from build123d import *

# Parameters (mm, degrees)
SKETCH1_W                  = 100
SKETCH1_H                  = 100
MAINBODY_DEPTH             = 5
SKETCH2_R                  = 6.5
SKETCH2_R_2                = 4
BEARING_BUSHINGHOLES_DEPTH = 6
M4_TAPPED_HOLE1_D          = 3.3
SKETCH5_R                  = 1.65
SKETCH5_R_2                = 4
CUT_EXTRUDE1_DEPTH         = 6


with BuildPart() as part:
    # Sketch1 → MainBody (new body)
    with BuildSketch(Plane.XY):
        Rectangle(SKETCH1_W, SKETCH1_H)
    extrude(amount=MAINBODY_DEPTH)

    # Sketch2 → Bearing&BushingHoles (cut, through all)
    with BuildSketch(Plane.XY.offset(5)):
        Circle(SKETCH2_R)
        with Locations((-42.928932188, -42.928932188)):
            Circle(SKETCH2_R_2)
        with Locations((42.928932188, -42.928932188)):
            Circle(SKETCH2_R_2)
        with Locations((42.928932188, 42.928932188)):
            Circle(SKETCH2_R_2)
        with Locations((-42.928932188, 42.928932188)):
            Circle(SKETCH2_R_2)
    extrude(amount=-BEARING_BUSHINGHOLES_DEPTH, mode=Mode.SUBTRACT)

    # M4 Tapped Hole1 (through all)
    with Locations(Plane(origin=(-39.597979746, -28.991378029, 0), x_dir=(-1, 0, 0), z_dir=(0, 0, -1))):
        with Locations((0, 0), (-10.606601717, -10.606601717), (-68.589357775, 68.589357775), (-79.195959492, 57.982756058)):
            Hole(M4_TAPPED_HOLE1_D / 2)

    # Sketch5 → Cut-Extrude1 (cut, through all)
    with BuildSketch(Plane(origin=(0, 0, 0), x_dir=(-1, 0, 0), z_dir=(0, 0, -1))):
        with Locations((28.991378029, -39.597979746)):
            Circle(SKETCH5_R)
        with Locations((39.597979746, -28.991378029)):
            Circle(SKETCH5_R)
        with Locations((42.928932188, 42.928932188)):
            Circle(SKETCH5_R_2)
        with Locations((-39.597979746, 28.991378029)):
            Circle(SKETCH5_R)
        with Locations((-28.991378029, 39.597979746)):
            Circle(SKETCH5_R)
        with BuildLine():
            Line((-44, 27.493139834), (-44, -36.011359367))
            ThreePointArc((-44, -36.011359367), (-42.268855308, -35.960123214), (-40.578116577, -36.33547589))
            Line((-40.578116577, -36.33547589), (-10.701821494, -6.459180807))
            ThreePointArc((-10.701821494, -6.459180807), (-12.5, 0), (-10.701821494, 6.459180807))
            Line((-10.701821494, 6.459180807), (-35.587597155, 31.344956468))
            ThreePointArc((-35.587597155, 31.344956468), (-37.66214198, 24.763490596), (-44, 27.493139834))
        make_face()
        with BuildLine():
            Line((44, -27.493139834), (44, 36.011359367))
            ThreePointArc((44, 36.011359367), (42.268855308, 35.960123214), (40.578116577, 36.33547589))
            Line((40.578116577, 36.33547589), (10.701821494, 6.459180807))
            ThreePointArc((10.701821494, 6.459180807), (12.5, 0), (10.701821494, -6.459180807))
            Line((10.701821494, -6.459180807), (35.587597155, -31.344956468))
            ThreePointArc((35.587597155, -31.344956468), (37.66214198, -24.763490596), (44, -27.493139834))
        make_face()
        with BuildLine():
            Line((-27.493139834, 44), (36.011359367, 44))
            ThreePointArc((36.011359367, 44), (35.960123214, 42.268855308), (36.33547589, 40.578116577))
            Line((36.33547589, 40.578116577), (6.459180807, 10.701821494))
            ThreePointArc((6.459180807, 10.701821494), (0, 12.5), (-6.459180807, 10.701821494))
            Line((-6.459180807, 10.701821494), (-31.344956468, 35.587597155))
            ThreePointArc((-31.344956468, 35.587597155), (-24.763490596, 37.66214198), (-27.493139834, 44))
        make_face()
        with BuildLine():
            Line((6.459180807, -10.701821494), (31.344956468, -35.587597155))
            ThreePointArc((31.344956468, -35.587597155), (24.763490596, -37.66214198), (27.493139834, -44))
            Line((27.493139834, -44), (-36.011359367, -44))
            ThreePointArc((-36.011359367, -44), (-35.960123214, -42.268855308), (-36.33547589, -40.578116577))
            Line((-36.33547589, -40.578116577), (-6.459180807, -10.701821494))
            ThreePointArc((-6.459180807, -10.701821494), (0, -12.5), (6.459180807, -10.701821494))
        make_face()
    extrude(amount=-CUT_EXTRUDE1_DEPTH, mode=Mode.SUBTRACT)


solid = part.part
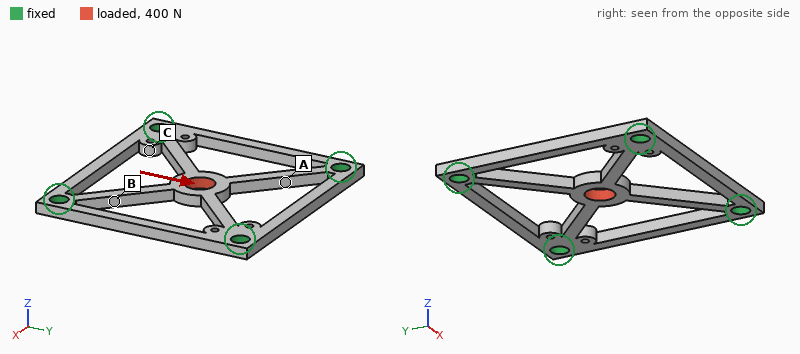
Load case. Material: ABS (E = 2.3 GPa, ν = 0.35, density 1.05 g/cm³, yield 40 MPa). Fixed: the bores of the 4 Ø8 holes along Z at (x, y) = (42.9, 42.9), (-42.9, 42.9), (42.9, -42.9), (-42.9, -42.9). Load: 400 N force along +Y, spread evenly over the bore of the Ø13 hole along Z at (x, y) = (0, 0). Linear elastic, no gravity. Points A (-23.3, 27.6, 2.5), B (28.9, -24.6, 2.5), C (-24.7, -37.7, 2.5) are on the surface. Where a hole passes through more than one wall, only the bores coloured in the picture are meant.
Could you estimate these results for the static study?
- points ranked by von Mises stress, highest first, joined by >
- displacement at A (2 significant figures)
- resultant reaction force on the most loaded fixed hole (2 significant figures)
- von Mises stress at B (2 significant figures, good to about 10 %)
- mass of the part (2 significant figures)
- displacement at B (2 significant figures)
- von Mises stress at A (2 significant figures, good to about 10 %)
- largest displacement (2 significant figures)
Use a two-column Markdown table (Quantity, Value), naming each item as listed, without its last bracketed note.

| Quantity | Value |
|---|---|
| points ranked by von Mises stress, highest first, joined by > | A > B > C |
| displacement at A | 0.061 mm |
| resultant reaction force on the most loaded fixed hole | 140 N |
| von Mises stress at B | 4.1 MPa |
| mass of the part | 21 g |
| displacement at B | 0.040 mm |
| von Mises stress at A | 5.0 MPa |
| largest displacement | 0.15 mm |
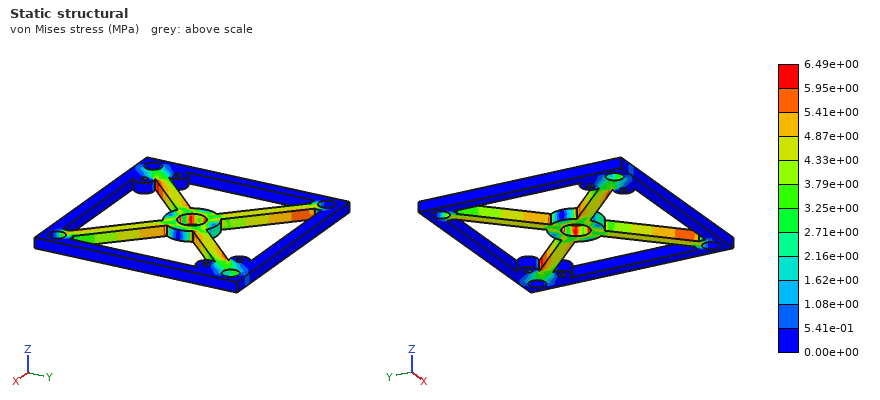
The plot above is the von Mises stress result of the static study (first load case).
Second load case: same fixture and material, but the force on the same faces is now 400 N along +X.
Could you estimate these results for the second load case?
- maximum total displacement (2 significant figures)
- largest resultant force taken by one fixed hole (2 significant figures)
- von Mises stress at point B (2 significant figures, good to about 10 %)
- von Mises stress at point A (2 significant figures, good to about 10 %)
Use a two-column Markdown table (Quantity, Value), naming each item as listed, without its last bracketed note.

| Quantity | Value |
|---|---|
| maximum total displacement | 0.15 mm |
| largest resultant force taken by one fixed hole | 140 N |
| von Mises stress at point B | 5.1 MPa |
| von Mises stress at point A | 4.2 MPa |
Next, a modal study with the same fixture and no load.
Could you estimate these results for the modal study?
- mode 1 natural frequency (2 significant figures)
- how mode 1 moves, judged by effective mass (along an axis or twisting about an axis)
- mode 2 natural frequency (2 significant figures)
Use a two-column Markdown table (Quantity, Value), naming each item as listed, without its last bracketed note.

| Quantity | Value |
|---|---|
| mode 1 natural frequency | 650 Hz |
| how mode 1 moves, judged by effective mass | along Z |
| mode 2 natural frequency | 1300 Hz |
